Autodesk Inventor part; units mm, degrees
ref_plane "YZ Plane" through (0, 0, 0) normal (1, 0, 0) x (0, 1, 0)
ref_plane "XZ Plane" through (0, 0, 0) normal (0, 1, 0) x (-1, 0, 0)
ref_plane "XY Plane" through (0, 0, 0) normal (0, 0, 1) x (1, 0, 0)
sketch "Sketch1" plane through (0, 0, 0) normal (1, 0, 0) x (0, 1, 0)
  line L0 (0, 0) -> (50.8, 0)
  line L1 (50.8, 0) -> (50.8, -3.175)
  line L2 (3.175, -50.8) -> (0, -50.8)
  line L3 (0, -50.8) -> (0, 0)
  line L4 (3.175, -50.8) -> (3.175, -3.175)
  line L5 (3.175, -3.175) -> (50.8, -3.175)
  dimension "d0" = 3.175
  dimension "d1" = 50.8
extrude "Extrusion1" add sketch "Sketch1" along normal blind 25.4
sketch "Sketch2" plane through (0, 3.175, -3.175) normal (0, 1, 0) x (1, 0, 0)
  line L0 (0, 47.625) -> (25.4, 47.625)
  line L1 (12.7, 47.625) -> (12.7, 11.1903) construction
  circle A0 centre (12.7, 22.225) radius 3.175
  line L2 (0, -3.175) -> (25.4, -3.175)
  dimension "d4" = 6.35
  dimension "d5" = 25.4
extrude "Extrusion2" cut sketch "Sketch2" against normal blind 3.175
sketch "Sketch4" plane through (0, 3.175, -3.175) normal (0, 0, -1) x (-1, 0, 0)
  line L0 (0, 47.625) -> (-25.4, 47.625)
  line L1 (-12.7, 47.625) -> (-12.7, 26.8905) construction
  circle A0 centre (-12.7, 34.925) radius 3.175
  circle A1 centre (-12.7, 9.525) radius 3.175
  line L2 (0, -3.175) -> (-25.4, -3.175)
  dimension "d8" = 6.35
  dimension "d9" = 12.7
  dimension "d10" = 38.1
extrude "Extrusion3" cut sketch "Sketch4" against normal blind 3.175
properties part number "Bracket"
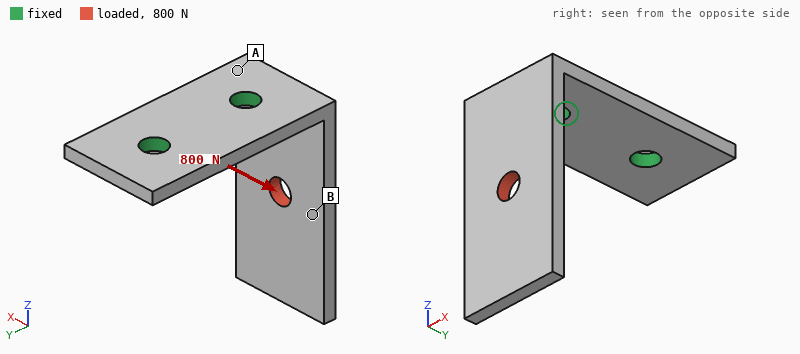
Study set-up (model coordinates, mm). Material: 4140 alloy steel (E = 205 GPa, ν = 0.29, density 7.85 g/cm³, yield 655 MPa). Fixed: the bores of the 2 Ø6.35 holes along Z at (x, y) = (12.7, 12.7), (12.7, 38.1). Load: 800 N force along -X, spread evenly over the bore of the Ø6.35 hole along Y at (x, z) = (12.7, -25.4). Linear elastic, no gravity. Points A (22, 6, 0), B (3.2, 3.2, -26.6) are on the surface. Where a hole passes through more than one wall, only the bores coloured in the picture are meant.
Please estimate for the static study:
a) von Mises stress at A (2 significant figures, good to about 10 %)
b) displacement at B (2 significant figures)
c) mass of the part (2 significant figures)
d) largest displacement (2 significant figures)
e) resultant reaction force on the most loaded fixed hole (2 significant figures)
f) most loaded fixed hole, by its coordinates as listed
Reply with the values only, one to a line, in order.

110 MPa
0.18 mm
60 g
0.33 mm
990 N
(12.7, 12.7)
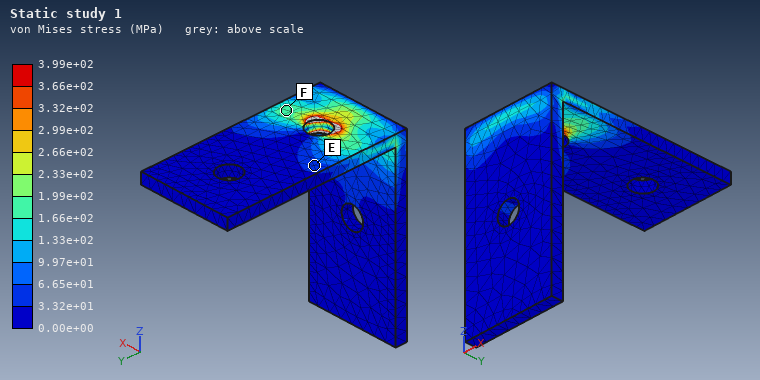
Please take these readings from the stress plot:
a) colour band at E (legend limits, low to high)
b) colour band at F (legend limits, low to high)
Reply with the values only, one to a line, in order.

3.32e+01 to 6.65e+01 MPa
1.66e+02 to 1.99e+02 MPa
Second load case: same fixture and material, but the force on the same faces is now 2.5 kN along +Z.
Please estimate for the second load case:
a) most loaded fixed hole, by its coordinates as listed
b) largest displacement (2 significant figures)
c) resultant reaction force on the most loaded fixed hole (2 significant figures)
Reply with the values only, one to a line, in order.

(12.7, 12.7)
0.44 mm
2.6 kN
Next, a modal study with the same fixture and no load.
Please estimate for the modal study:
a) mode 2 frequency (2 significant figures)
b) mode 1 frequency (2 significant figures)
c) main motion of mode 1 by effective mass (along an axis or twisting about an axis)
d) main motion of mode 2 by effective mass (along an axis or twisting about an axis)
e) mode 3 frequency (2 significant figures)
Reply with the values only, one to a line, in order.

1700 Hz
830 Hz
along Y
along X
4100 Hz
